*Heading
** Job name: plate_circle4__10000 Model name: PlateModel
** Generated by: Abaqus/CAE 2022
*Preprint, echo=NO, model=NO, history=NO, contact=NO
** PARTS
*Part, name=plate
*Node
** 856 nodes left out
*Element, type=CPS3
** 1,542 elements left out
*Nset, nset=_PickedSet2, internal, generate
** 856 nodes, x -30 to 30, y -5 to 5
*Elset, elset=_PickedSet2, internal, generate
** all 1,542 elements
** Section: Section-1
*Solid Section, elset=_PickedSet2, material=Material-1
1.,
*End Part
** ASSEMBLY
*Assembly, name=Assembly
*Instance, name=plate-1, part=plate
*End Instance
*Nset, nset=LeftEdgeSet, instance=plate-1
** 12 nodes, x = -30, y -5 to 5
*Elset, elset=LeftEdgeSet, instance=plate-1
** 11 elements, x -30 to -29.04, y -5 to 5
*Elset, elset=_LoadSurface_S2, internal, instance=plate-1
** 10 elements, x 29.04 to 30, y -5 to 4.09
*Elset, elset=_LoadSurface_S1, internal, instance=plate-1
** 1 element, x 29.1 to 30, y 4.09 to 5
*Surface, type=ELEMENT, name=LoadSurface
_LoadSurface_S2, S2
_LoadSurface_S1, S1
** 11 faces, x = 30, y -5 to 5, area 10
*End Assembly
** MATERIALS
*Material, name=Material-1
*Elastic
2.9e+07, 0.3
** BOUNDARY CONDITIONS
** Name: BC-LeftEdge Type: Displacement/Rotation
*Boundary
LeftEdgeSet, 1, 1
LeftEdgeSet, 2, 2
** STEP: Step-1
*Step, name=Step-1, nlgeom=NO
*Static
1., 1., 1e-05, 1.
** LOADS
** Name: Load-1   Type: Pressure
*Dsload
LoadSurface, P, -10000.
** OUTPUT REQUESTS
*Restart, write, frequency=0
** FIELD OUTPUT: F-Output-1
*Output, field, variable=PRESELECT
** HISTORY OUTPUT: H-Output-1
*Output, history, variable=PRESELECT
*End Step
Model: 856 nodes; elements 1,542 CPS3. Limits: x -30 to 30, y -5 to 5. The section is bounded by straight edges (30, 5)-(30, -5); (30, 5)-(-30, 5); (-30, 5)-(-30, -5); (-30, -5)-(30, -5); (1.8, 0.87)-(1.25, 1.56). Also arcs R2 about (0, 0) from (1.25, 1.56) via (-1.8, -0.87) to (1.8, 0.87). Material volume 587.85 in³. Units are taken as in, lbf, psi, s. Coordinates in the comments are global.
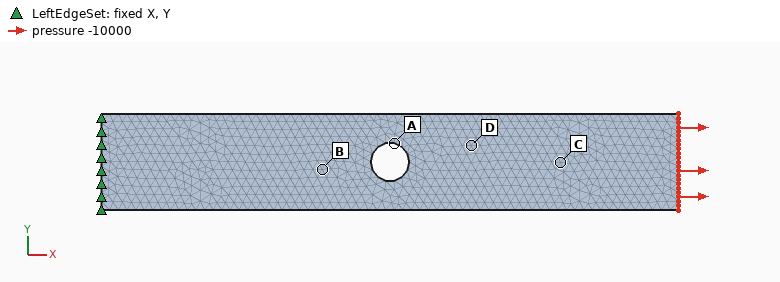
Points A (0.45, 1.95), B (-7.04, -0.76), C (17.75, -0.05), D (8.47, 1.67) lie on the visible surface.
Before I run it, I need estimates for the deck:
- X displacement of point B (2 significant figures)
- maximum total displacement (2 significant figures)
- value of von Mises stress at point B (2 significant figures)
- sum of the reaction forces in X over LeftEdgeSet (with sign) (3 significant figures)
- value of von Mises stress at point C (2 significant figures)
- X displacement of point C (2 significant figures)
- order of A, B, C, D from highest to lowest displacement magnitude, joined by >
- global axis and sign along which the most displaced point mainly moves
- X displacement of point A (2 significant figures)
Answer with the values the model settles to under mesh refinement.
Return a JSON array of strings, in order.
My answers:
["0.0078 in", "0.022 in", "8300 psi", "-1.00e+05 lbf", "10000 psi", "0.018 in", "C > D > A > B", "+X", "0.012 in"]
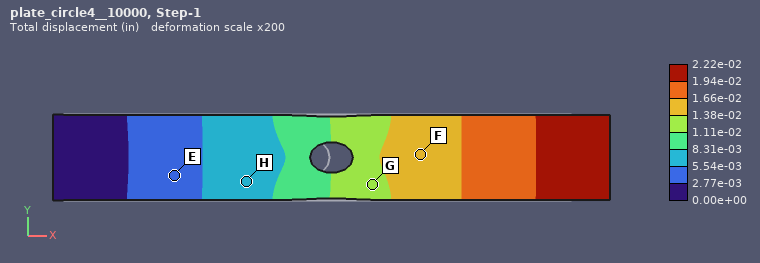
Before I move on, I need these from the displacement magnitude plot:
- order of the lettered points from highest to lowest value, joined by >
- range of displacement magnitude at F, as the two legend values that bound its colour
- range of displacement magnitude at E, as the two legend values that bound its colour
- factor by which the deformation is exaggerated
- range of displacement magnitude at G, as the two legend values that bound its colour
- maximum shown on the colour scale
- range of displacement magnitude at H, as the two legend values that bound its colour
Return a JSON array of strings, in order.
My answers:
["F > G > H > E", "1.38e-02 to 1.66e-02 in", "2.77e-03 to 5.54e-03 in", "200", "1.11e-02 to 1.38e-02 in", "2.22e-02 in", "5.54e-03 to 8.31e-03 in"]
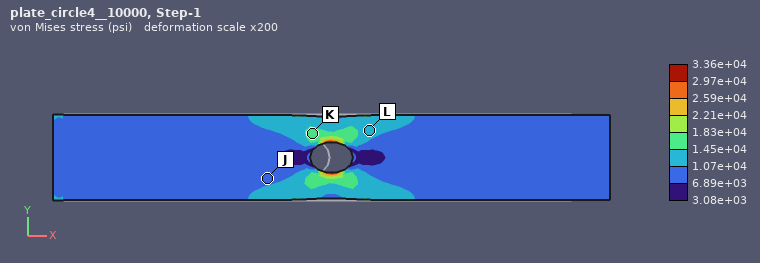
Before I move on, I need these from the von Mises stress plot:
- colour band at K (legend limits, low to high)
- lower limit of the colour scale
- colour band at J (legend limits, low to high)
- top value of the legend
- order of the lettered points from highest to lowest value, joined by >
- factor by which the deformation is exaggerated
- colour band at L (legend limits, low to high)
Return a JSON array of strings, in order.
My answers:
["1.45e+04 to 1.83e+04 psi", "3.08e+03 psi", "6.89e+03 to 1.07e+04 psi", "3.36e+04 psi", "K > L > J", "200", "1.07e+04 to 1.45e+04 psi"]
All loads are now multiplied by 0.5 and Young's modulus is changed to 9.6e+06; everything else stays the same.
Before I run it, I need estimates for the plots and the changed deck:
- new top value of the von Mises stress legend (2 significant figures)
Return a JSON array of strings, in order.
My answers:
["17000 psi"]
